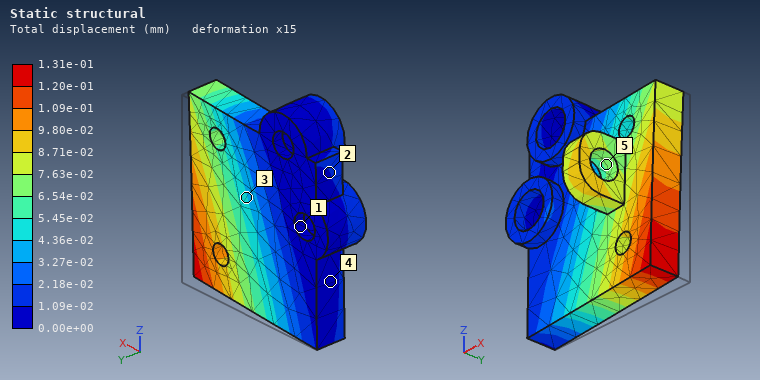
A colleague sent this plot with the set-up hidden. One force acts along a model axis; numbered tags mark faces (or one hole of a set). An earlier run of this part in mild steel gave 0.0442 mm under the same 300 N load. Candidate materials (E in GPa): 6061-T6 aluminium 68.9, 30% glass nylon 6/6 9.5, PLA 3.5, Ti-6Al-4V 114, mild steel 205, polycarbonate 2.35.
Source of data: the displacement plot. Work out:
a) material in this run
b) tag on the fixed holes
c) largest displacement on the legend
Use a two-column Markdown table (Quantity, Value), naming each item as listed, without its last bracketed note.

| Quantity | Value |
|---|---|
| material in this run | 6061-T6 aluminium |
| tag on the fixed holes | 1 |
| largest displacement on the legend | 1.31e-01 mm |
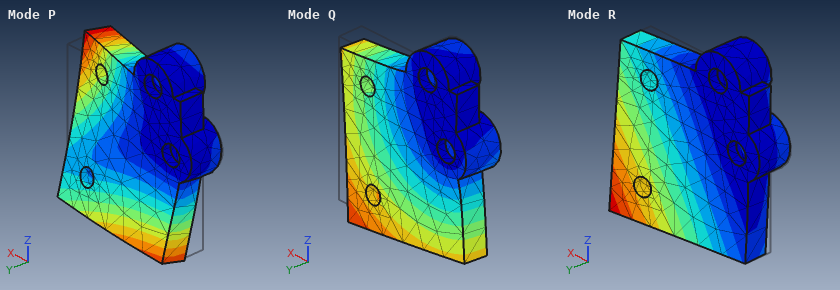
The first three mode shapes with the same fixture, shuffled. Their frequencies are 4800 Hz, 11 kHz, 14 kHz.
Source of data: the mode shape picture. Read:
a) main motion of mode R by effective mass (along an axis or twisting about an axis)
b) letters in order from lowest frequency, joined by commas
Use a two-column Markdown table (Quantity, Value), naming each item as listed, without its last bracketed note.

| Quantity | Value |
|---|---|
| main motion of mode R by effective mass | along Y |
| letters in order from lowest frequency, joined by commas | R, P, Q |
